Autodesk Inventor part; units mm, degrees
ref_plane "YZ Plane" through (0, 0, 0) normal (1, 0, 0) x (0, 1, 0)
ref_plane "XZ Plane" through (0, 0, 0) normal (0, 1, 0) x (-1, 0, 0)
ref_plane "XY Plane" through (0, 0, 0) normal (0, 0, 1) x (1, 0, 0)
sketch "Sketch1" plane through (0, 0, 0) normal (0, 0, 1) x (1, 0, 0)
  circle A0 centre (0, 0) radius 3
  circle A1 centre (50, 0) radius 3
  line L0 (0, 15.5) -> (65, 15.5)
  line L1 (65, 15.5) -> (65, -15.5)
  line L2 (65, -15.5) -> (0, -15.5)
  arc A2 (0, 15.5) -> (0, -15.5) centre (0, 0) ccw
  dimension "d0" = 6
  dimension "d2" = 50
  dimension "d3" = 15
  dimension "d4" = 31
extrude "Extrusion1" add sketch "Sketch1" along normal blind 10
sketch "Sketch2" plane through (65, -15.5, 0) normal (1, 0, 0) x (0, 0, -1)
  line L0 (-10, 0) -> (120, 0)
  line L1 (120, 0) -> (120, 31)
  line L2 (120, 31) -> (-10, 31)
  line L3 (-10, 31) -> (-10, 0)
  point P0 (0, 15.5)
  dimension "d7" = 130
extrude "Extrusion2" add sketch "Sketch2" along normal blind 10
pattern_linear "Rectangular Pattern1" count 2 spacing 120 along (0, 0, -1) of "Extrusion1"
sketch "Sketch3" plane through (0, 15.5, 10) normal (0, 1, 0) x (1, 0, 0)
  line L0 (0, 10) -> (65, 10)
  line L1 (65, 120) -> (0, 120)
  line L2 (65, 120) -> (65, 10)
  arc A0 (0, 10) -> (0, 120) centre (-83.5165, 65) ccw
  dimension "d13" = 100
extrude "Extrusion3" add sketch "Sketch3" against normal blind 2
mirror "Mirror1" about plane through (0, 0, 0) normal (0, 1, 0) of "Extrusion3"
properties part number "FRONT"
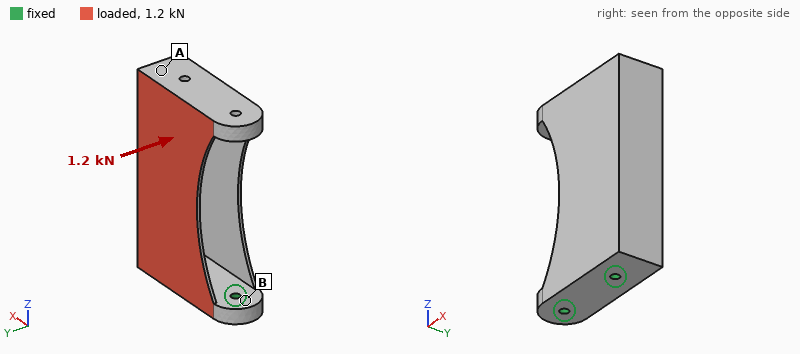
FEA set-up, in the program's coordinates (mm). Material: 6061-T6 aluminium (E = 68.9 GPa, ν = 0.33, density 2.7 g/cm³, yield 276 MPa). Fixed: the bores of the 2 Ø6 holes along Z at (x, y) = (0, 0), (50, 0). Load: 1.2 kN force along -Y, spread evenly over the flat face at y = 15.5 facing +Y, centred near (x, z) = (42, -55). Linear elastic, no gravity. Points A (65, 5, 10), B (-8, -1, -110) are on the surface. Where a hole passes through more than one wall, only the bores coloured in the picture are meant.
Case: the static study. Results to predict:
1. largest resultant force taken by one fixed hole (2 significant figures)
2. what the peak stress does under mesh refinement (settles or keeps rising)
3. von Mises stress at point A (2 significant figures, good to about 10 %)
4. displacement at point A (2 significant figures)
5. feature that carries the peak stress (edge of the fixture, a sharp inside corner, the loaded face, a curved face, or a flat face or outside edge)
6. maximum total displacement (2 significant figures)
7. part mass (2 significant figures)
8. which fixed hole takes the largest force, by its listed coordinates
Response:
980 N
keeps rising
20 MPa
0.53 mm
edge of the fixture
1.1 mm
300 g
(50, 0)
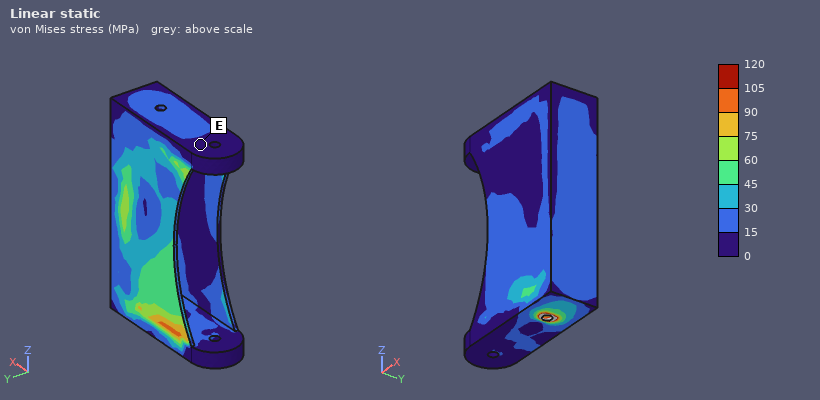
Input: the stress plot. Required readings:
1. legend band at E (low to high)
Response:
0 to 15 MPa
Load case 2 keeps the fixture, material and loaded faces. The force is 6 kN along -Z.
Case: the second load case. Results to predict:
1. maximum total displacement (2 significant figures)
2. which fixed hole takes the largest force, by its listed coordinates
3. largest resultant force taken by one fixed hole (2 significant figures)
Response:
0.47 mm
(50, 0)
4.7 kN
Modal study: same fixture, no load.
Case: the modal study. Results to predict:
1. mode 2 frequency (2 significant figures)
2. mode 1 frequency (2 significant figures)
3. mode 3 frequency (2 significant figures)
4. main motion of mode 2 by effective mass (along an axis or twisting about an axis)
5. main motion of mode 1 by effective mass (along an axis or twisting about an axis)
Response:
1200 Hz
400 Hz
1500 Hz
along X
along Y
